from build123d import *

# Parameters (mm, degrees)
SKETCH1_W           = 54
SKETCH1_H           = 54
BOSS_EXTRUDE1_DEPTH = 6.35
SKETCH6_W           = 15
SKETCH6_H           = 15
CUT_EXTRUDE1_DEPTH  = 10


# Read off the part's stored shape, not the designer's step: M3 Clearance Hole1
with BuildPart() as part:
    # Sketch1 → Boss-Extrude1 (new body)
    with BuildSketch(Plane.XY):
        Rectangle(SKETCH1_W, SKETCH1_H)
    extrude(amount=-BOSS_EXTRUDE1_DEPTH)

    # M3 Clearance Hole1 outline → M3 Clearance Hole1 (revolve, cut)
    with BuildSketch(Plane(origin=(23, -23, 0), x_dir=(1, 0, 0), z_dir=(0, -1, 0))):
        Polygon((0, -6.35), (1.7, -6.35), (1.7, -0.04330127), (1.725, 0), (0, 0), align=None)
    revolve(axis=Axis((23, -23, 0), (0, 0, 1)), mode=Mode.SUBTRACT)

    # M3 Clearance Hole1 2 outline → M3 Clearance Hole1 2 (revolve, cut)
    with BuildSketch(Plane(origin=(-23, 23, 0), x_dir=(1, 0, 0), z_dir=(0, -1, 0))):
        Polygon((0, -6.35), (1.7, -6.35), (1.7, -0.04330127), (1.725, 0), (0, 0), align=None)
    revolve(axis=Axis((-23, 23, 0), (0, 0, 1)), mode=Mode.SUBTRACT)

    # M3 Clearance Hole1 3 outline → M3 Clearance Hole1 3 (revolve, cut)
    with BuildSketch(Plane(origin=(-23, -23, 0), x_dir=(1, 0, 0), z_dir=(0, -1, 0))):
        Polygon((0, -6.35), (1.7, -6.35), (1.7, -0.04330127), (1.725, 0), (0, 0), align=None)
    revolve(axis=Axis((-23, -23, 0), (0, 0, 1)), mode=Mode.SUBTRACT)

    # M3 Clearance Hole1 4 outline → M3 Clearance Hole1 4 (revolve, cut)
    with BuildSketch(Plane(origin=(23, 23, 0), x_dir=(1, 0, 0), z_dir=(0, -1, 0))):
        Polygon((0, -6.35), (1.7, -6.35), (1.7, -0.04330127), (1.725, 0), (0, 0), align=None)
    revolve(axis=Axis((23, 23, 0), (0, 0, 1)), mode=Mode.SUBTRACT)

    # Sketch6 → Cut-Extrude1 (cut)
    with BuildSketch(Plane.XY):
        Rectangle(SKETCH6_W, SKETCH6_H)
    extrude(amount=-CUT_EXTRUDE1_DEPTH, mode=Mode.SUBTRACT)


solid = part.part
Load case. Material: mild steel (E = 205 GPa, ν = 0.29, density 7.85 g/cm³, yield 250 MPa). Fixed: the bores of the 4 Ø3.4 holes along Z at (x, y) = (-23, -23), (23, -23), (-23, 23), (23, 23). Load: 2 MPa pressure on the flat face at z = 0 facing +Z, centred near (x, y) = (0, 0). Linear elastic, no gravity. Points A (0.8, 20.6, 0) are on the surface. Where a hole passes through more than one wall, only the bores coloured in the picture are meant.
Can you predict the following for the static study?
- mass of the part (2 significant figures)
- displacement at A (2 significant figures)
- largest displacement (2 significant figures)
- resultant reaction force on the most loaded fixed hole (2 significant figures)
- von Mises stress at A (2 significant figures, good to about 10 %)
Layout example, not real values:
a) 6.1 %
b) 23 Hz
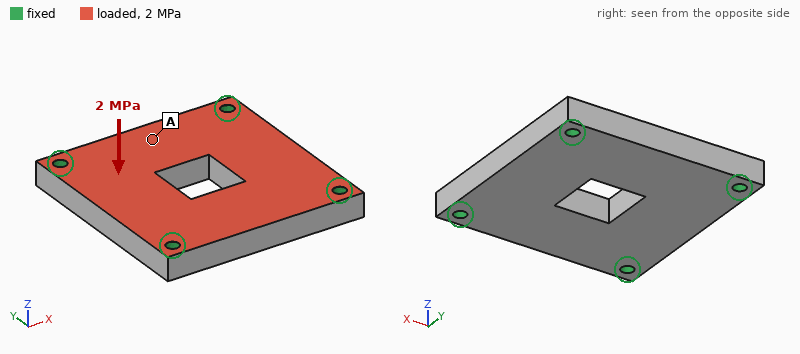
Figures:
a) 130 g
b) 11 µm
c) 18 µm
d) 1.3 kN
e) 34 MPa
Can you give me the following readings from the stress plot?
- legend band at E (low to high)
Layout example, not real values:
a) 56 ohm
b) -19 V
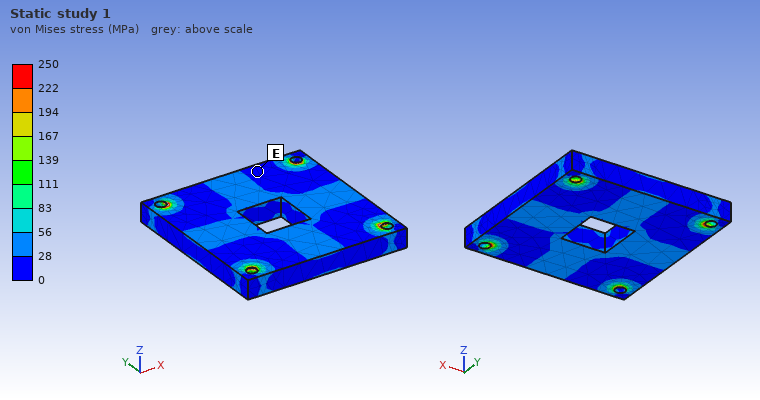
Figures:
a) 0 to 28 MPa
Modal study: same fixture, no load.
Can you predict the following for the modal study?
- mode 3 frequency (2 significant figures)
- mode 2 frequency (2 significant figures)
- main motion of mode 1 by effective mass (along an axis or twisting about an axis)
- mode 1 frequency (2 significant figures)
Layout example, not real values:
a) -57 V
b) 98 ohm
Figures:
a) 15 kHz
b) 15 kHz
c) along Z
d) 9300 Hz
